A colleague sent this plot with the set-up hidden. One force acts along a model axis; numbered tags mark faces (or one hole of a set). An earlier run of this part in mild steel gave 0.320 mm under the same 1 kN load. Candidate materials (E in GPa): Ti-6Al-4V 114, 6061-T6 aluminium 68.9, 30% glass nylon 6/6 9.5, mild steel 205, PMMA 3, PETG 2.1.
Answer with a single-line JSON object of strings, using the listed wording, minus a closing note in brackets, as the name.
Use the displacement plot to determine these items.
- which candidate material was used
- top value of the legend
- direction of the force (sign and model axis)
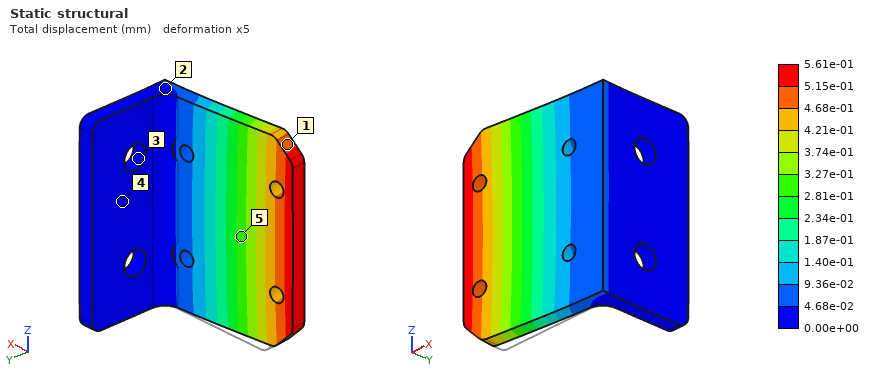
{"which candidate material was used": "Ti-6Al-4V", "top value of the legend": "5.61e-01 mm", "direction of the force": "-Y"}
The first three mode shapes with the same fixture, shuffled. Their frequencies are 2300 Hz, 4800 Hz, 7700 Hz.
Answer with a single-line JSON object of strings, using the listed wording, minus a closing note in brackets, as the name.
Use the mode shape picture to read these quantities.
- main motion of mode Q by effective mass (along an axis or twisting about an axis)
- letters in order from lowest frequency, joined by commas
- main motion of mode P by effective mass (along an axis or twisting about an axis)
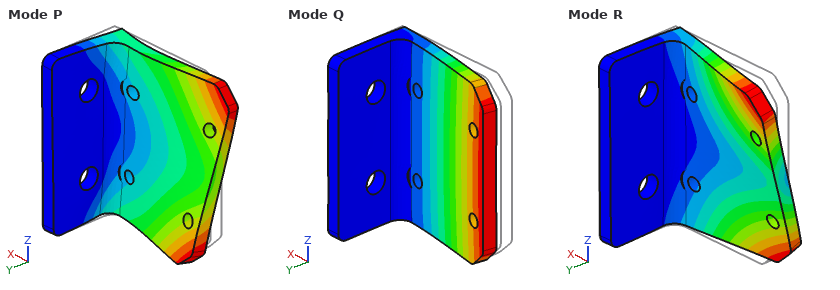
{"main motion of mode Q by effective mass": "along Y", "letters in order from lowest frequency, joined by commas": "Q, R, P", "main motion of mode P by effective mass": "along Z"}
